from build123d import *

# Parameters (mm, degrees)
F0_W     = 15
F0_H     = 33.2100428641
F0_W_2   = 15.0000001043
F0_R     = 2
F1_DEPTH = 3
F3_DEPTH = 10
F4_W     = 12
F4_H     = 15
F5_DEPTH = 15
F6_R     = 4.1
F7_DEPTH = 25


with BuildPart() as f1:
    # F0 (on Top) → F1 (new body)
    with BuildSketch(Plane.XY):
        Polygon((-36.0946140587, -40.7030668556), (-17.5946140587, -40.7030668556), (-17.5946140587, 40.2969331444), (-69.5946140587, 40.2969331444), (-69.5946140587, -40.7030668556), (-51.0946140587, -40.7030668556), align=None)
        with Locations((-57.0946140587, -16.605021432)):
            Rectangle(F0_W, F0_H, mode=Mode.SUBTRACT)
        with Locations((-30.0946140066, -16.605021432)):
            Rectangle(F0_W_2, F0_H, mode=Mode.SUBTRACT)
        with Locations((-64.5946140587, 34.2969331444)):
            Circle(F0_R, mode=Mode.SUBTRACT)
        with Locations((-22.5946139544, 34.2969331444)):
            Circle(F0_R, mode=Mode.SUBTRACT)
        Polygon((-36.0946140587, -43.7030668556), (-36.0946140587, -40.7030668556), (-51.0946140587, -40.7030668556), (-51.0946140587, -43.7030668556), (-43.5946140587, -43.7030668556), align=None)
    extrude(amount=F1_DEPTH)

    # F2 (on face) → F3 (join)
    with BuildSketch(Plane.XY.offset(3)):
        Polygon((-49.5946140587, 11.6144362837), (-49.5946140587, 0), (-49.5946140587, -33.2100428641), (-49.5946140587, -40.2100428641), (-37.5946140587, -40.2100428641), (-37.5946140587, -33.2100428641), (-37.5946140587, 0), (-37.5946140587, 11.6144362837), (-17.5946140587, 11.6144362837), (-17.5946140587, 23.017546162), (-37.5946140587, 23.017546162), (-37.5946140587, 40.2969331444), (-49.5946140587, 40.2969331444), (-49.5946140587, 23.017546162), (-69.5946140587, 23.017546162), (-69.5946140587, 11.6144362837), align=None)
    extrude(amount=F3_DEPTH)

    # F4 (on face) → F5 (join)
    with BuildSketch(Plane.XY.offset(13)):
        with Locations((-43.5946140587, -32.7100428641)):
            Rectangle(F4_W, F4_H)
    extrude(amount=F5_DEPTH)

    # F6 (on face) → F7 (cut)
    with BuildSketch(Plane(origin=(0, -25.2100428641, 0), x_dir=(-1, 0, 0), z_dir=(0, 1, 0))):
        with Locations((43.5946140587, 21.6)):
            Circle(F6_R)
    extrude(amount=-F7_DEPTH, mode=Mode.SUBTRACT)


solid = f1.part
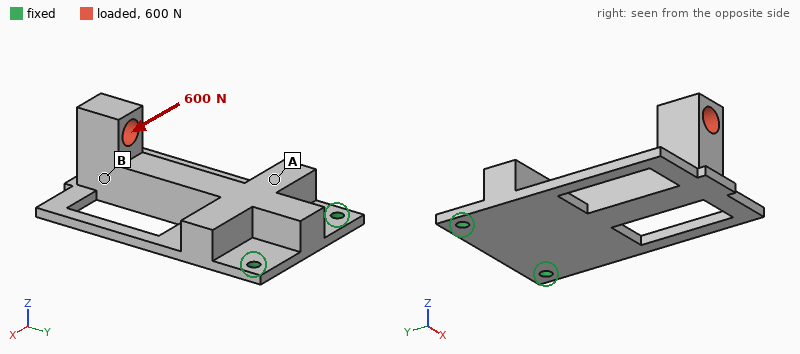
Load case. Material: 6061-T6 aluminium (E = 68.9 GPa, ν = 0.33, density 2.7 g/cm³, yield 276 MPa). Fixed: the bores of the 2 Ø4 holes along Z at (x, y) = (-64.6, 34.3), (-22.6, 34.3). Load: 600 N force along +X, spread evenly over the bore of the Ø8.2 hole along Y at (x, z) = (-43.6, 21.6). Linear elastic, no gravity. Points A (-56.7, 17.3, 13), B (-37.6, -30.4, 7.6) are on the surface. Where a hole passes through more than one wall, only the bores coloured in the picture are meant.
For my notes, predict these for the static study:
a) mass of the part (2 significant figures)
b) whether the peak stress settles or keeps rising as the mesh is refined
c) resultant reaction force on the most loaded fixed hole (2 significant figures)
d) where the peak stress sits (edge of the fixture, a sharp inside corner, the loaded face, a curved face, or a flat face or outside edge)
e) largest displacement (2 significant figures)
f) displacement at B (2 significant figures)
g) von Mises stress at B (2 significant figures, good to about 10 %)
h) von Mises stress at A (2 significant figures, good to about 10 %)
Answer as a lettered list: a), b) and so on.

a) 70 g
b) keeps rising
c) 1.0 kN
d) edge of the fixture
e) 0.26 mm
f) 0.11 mm
g) 28 MPa
h) 12 MPa
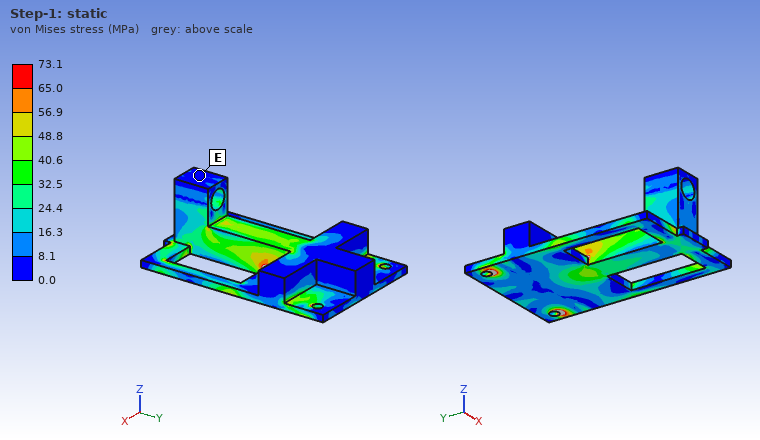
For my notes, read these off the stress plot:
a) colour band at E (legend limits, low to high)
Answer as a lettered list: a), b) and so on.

a) 0.0 to 8.1 MPa
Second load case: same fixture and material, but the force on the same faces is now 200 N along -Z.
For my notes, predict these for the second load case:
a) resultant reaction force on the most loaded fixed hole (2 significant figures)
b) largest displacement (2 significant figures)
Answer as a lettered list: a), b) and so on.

a) 120 N
b) 1.1 mm
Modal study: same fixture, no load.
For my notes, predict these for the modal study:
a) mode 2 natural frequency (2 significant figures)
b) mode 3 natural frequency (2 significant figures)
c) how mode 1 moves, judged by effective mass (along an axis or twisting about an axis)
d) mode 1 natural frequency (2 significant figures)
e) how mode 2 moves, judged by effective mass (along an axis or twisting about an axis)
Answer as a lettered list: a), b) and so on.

a) 2700 Hz
b) 3300 Hz
c) along Z
d) 470 Hz
e) along X
